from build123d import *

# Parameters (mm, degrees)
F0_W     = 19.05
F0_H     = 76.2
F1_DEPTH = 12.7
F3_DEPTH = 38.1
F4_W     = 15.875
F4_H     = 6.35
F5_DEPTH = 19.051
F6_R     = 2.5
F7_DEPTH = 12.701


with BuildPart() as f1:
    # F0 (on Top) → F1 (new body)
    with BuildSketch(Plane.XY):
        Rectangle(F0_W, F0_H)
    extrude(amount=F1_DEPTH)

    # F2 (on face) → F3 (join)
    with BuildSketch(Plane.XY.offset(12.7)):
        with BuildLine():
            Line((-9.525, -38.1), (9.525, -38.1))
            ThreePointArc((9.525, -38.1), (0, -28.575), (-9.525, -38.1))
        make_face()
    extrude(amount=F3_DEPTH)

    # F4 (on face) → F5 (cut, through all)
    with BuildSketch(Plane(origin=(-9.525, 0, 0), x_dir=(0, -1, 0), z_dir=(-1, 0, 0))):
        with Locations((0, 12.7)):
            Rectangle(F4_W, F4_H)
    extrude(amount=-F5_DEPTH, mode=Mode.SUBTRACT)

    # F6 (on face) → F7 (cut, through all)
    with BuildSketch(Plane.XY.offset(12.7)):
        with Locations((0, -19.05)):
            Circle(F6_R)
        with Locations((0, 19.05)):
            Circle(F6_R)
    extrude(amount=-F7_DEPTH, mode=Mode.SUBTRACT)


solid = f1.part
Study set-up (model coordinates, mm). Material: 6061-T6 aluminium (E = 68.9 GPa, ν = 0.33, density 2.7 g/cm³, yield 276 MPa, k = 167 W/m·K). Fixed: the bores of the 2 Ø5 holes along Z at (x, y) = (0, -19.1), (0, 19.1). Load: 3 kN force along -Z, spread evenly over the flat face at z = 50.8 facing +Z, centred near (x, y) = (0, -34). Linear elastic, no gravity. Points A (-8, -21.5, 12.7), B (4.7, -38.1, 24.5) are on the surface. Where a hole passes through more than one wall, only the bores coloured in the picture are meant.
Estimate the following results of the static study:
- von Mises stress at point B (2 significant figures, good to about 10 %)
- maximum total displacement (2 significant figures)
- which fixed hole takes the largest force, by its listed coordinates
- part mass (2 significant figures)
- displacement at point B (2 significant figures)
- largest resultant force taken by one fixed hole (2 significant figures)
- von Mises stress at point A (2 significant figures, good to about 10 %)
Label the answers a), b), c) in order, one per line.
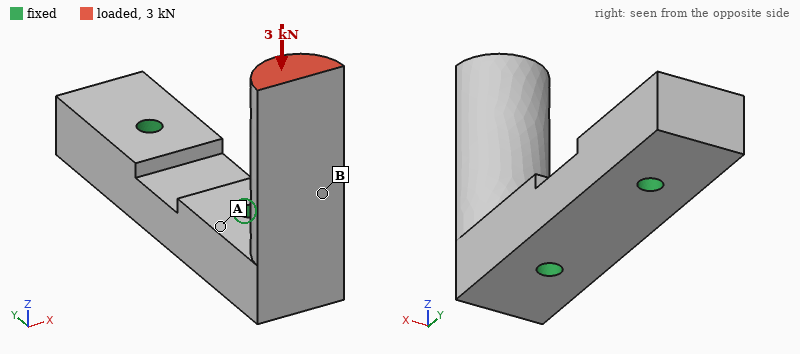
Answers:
a) 21 MPa
b) 96 µm
c) (0, -19.1)
d) 60 g
e) 50 µm
f) 3.2 kN
g) 41 MPa
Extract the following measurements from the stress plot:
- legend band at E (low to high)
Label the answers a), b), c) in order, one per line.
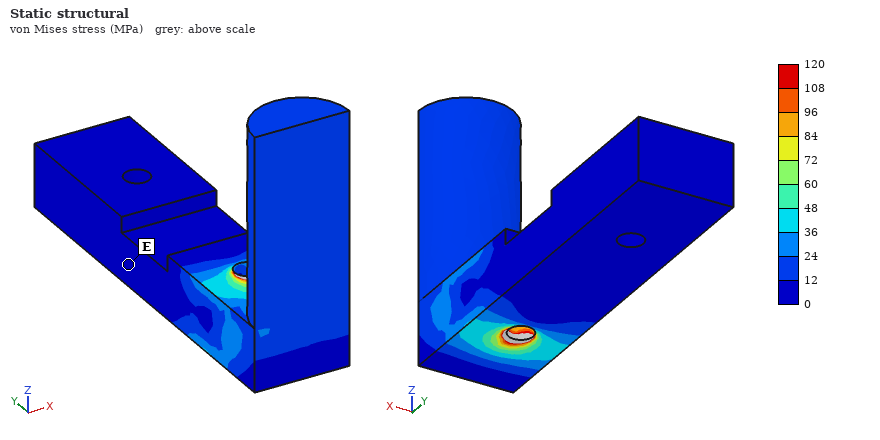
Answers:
a) 0 to 12 MPa
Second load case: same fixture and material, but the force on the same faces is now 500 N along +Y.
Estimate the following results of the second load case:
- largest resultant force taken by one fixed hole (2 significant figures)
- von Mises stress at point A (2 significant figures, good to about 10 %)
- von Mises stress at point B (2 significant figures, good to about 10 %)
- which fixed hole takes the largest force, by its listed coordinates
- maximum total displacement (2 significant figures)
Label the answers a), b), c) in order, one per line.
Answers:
a) 540 N
b) 26 MPa
c) 59 MPa
d) (0, -19.1)
e) 0.26 mm
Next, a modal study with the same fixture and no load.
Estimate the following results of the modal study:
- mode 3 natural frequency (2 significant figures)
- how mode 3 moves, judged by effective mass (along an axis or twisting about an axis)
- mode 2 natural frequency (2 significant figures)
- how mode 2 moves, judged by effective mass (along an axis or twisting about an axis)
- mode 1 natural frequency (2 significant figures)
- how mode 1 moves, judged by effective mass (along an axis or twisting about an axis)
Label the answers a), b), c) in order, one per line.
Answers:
a) 12 kHz
b) along Z
c) 4300 Hz
d) along X
e) 3400 Hz
f) along Y
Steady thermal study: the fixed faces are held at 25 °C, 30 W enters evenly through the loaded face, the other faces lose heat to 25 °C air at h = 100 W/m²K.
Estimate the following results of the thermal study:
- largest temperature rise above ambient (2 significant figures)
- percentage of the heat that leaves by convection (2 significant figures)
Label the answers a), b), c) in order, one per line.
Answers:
a) 53 K
b) 22 %
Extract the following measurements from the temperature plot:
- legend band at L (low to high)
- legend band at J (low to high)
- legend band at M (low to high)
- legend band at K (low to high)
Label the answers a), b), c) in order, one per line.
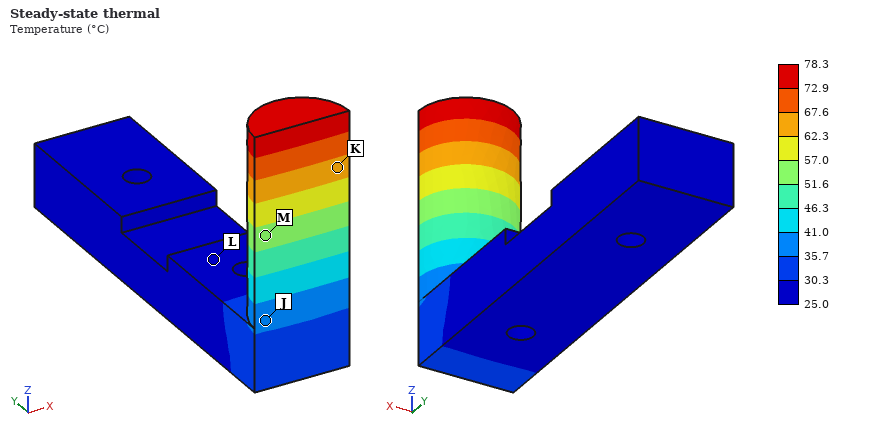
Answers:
a) 25.0 to 30.3 °C
b) 35.7 to 41.0 °C
c) 51.6 to 57.0 °C
d) 62.3 to 67.6 °C
